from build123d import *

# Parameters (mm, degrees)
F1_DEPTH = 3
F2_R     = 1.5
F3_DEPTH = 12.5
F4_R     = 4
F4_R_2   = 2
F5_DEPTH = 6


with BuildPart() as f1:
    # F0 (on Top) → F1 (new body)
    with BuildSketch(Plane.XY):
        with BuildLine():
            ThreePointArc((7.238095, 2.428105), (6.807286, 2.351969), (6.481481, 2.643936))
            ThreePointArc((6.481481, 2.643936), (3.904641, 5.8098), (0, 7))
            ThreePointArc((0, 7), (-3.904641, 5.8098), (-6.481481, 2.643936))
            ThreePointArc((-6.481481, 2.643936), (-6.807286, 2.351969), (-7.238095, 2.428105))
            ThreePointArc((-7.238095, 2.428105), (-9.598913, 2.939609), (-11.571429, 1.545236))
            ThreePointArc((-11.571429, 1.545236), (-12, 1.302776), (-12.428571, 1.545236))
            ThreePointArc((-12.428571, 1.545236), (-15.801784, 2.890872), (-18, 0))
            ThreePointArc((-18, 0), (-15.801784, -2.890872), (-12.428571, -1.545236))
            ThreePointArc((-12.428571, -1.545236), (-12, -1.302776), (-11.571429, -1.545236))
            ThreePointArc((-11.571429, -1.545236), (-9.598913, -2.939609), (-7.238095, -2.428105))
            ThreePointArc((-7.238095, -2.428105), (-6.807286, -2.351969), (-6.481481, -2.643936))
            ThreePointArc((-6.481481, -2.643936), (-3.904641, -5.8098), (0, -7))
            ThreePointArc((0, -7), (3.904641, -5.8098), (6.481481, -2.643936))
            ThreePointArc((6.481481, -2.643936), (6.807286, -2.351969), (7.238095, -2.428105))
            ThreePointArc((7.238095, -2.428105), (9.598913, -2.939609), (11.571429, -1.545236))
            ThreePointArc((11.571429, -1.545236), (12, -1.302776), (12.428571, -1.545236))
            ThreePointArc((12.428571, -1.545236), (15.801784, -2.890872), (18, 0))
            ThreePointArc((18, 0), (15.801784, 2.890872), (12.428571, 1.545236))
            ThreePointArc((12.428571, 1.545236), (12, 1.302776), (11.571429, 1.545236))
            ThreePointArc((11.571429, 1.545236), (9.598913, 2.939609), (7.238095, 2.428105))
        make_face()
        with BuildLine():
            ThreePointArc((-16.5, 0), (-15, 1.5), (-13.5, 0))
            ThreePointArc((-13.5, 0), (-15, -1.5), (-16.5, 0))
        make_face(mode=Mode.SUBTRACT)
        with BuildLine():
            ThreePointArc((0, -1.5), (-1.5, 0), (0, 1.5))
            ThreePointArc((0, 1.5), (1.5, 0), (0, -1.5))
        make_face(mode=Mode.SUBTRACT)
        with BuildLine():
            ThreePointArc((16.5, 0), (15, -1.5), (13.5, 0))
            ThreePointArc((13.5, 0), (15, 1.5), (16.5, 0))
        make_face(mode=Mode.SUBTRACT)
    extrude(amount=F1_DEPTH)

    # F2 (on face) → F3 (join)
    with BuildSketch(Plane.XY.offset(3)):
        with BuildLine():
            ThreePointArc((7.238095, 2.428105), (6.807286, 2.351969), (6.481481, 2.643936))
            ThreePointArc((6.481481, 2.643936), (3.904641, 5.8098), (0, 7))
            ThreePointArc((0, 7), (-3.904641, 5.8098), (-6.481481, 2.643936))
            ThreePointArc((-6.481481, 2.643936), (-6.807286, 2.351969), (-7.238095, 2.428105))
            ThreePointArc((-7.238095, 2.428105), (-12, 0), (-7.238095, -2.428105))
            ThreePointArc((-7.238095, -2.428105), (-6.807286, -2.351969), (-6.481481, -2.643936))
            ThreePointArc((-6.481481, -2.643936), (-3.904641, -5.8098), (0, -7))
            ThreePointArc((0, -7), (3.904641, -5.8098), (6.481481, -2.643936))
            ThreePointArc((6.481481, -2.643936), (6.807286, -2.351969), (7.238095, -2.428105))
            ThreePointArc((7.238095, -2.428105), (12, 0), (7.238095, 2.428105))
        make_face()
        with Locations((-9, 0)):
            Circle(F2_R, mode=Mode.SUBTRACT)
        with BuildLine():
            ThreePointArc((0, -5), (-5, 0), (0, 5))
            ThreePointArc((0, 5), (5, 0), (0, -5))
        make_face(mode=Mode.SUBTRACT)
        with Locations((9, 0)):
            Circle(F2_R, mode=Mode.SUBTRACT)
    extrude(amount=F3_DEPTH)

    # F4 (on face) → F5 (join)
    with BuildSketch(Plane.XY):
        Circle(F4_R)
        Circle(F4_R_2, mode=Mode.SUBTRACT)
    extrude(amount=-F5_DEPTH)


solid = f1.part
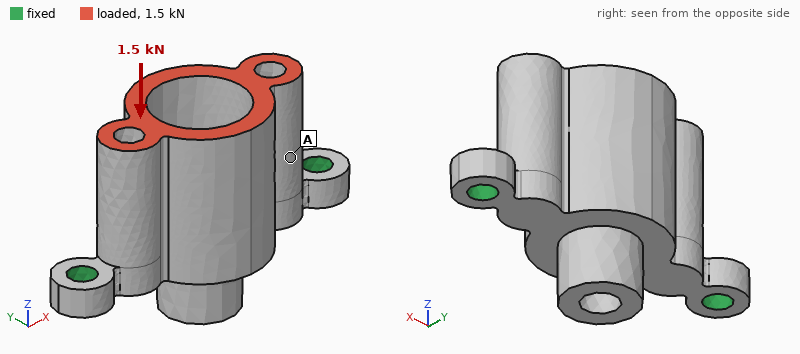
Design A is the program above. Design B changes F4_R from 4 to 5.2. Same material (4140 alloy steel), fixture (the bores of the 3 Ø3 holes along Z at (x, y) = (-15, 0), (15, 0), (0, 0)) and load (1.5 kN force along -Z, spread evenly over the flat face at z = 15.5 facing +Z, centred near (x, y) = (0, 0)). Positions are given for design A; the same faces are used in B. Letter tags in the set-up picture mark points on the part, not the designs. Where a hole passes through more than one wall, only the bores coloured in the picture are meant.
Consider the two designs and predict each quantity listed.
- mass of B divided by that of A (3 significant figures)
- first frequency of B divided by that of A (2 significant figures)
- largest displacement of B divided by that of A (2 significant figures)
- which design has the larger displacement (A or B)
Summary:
1.09
1.0
0.87
A
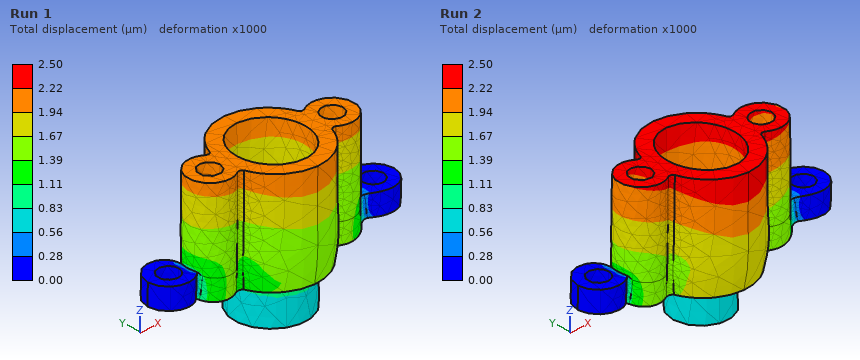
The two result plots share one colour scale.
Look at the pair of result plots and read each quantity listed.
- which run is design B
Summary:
Run 1
